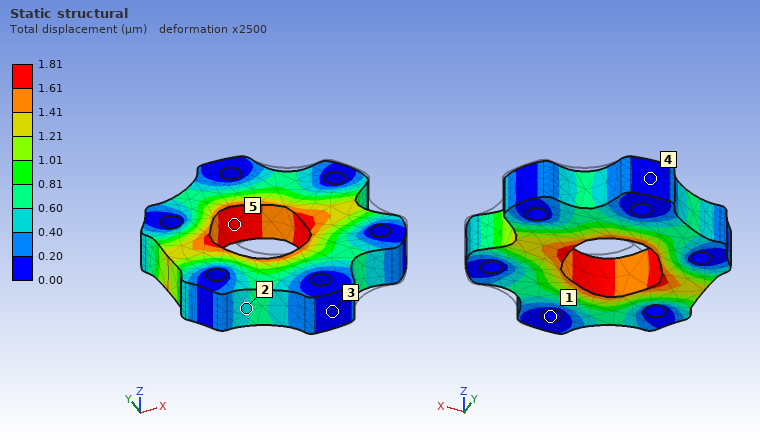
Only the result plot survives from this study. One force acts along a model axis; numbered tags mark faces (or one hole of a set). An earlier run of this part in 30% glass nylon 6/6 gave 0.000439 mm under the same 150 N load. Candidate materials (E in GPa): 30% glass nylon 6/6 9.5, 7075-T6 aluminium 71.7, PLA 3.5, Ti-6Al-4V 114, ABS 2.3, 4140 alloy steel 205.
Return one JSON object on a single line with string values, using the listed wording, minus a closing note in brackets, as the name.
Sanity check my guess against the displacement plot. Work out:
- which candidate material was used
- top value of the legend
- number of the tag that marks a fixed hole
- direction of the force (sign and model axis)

{"which candidate material was used": "ABS", "top value of the legend": "1.81 µm", "number of the tag that marks a fixed hole": "1", "direction of the force": "-X"}
